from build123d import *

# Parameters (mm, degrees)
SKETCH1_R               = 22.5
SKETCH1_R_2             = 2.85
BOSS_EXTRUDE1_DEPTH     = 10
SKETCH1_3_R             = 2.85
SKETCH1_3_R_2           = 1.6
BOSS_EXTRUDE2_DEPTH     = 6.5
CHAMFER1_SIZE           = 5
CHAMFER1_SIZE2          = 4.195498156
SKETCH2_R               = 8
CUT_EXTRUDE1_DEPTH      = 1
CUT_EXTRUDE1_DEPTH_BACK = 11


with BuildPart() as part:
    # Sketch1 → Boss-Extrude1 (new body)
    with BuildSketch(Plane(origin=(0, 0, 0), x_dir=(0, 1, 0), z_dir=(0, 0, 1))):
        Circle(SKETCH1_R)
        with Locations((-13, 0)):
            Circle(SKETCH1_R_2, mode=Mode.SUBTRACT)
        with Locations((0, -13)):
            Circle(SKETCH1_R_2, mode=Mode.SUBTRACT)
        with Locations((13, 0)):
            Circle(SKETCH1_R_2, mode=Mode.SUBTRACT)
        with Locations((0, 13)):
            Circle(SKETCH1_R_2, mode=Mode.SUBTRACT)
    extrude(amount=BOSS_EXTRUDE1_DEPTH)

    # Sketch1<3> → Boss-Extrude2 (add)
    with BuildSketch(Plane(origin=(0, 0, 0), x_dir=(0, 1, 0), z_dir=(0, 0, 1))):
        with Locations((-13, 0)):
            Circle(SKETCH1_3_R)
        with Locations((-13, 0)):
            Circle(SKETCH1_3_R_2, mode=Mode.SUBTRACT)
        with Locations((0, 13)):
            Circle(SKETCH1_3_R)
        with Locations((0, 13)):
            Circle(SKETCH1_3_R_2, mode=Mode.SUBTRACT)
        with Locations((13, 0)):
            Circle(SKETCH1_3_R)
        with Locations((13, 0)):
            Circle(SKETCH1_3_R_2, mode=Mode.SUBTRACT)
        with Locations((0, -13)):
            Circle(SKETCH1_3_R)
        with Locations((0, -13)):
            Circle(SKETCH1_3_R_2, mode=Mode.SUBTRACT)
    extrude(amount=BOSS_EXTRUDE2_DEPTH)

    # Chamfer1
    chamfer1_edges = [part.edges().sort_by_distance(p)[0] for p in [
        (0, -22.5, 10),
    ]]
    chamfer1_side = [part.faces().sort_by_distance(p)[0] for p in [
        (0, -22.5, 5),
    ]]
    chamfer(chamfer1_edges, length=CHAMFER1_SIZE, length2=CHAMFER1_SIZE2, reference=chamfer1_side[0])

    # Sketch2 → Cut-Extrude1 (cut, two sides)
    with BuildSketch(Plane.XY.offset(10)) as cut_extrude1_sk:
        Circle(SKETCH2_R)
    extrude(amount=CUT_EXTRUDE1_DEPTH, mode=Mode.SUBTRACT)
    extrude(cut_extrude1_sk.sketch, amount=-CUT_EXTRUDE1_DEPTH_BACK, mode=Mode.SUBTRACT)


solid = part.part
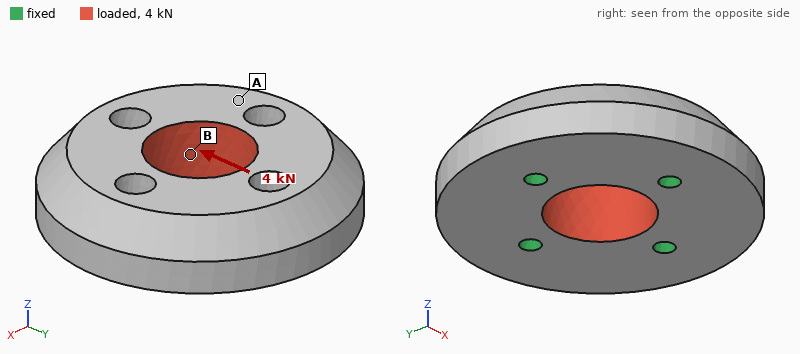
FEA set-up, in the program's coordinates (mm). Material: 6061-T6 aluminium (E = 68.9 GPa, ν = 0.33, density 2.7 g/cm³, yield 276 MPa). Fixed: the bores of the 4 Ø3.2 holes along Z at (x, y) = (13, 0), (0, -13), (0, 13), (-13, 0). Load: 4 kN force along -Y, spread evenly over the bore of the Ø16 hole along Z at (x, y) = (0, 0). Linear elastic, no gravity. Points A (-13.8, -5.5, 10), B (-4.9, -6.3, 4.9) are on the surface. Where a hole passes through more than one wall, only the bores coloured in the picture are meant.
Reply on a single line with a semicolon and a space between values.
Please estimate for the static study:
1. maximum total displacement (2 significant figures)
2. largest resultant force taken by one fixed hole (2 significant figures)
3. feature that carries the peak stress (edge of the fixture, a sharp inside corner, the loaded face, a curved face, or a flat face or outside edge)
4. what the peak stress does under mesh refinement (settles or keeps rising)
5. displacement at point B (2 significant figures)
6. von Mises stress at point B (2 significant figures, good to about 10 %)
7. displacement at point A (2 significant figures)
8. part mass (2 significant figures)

3.0 µm; 1.0 kN; edge of the fixture; keeps rising; 1.7 µm; 12 MPa; 1.2 µm; 32 g
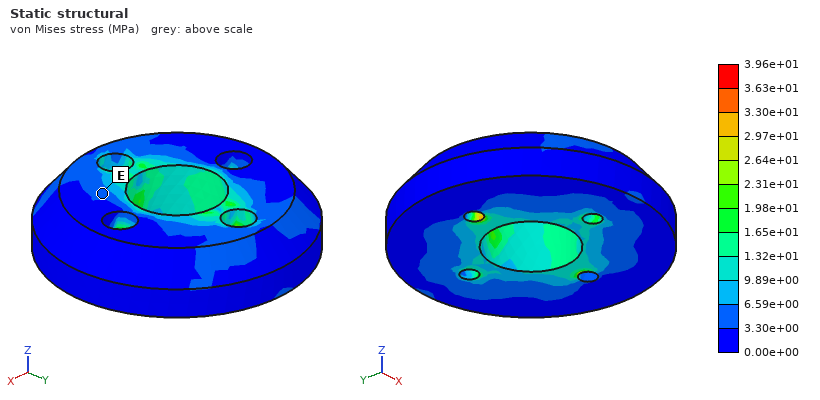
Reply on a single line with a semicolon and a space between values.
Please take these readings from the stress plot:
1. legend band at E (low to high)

3.30e+00 to 6.59e+00 MPa
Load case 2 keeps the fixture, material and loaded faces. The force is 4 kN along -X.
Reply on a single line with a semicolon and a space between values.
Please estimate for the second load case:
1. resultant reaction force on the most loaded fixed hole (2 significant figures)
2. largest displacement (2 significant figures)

1.0 kN; 3.0 µm
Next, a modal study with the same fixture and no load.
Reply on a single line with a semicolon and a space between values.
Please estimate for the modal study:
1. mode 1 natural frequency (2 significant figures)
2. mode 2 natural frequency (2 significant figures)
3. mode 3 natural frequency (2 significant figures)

27 kHz; 29 kHz; 29 kHz
